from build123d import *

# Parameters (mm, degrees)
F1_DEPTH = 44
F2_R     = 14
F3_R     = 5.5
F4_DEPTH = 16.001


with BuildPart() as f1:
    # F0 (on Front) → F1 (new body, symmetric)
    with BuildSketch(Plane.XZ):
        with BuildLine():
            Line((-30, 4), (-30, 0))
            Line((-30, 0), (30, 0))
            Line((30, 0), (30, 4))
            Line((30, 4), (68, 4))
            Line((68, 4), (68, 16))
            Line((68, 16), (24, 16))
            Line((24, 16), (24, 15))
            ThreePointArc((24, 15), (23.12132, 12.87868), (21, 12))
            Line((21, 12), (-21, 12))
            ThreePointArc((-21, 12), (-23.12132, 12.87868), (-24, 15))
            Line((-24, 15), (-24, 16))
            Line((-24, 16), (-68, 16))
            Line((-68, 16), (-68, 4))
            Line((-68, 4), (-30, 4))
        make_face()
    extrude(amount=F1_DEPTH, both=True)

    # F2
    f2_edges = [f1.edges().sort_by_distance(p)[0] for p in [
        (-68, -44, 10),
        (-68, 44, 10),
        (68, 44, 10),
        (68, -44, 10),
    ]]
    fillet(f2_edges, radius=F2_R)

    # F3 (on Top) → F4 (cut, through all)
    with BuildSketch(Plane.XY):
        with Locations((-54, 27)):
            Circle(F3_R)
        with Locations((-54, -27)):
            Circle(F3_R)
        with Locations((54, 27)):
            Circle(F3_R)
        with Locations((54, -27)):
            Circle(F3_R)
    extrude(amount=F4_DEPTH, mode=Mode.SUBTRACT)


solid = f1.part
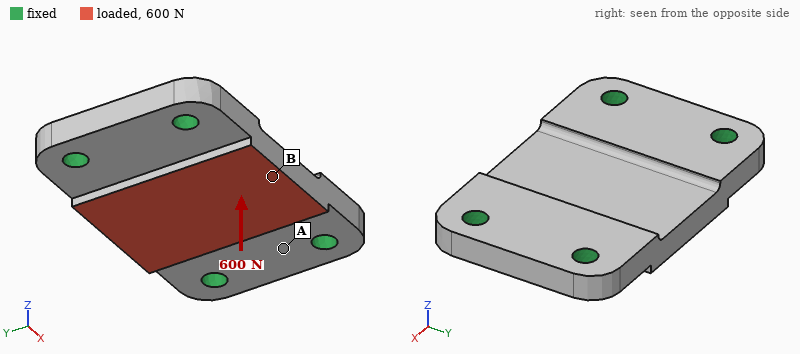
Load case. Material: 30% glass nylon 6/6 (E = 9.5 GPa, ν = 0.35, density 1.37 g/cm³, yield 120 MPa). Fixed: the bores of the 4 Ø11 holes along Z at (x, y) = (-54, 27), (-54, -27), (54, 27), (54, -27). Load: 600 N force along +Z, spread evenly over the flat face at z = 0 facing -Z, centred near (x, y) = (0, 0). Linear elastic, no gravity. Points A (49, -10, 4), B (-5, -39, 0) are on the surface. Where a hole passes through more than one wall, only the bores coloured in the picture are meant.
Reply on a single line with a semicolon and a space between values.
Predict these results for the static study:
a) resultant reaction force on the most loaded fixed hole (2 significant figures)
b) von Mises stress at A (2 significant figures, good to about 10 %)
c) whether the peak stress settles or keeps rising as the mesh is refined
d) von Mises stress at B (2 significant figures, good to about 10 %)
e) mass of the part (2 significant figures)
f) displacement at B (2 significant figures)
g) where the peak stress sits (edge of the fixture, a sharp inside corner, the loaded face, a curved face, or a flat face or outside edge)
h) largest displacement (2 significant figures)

240 N; 0.78 MPa; keeps rising; 2.0 MPa; 190 g; 23 µm; edge of the fixture; 24 µm
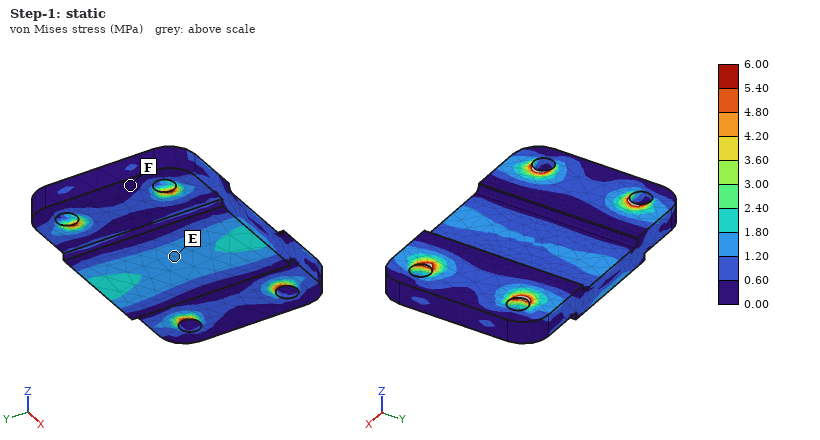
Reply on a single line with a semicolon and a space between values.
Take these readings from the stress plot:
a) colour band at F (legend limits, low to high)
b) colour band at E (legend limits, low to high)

0.00 to 0.60 MPa; 1.20 to 1.80 MPa
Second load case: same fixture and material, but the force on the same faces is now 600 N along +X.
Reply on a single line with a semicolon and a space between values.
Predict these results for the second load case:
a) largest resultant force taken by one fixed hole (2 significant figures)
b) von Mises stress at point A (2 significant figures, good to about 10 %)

160 N; 0.16 MPa
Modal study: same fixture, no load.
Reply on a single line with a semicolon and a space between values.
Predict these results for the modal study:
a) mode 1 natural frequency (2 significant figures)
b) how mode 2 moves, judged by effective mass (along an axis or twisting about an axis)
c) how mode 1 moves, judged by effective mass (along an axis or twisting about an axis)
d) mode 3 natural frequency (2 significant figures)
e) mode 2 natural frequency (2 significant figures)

2800 Hz; twisting about X; along Z; 6100 Hz; 3500 Hz
